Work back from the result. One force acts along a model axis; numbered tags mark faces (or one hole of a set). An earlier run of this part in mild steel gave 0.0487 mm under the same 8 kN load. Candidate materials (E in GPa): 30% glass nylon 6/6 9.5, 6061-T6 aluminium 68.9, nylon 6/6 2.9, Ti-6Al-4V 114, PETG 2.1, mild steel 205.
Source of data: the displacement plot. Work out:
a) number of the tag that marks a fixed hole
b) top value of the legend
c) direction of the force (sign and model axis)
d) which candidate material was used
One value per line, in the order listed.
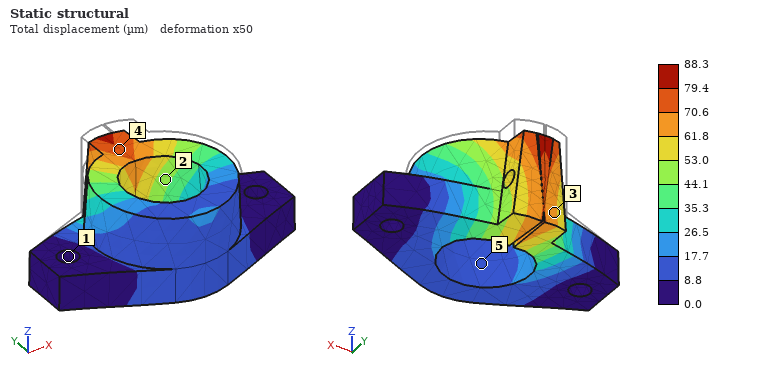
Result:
1
88.3 µm
-Z
Ti-6Al-4V
